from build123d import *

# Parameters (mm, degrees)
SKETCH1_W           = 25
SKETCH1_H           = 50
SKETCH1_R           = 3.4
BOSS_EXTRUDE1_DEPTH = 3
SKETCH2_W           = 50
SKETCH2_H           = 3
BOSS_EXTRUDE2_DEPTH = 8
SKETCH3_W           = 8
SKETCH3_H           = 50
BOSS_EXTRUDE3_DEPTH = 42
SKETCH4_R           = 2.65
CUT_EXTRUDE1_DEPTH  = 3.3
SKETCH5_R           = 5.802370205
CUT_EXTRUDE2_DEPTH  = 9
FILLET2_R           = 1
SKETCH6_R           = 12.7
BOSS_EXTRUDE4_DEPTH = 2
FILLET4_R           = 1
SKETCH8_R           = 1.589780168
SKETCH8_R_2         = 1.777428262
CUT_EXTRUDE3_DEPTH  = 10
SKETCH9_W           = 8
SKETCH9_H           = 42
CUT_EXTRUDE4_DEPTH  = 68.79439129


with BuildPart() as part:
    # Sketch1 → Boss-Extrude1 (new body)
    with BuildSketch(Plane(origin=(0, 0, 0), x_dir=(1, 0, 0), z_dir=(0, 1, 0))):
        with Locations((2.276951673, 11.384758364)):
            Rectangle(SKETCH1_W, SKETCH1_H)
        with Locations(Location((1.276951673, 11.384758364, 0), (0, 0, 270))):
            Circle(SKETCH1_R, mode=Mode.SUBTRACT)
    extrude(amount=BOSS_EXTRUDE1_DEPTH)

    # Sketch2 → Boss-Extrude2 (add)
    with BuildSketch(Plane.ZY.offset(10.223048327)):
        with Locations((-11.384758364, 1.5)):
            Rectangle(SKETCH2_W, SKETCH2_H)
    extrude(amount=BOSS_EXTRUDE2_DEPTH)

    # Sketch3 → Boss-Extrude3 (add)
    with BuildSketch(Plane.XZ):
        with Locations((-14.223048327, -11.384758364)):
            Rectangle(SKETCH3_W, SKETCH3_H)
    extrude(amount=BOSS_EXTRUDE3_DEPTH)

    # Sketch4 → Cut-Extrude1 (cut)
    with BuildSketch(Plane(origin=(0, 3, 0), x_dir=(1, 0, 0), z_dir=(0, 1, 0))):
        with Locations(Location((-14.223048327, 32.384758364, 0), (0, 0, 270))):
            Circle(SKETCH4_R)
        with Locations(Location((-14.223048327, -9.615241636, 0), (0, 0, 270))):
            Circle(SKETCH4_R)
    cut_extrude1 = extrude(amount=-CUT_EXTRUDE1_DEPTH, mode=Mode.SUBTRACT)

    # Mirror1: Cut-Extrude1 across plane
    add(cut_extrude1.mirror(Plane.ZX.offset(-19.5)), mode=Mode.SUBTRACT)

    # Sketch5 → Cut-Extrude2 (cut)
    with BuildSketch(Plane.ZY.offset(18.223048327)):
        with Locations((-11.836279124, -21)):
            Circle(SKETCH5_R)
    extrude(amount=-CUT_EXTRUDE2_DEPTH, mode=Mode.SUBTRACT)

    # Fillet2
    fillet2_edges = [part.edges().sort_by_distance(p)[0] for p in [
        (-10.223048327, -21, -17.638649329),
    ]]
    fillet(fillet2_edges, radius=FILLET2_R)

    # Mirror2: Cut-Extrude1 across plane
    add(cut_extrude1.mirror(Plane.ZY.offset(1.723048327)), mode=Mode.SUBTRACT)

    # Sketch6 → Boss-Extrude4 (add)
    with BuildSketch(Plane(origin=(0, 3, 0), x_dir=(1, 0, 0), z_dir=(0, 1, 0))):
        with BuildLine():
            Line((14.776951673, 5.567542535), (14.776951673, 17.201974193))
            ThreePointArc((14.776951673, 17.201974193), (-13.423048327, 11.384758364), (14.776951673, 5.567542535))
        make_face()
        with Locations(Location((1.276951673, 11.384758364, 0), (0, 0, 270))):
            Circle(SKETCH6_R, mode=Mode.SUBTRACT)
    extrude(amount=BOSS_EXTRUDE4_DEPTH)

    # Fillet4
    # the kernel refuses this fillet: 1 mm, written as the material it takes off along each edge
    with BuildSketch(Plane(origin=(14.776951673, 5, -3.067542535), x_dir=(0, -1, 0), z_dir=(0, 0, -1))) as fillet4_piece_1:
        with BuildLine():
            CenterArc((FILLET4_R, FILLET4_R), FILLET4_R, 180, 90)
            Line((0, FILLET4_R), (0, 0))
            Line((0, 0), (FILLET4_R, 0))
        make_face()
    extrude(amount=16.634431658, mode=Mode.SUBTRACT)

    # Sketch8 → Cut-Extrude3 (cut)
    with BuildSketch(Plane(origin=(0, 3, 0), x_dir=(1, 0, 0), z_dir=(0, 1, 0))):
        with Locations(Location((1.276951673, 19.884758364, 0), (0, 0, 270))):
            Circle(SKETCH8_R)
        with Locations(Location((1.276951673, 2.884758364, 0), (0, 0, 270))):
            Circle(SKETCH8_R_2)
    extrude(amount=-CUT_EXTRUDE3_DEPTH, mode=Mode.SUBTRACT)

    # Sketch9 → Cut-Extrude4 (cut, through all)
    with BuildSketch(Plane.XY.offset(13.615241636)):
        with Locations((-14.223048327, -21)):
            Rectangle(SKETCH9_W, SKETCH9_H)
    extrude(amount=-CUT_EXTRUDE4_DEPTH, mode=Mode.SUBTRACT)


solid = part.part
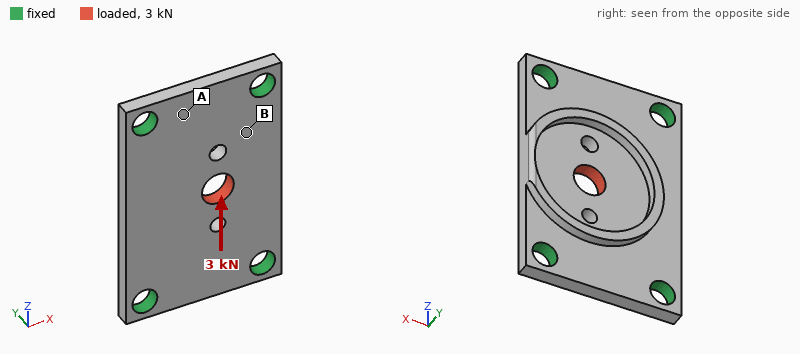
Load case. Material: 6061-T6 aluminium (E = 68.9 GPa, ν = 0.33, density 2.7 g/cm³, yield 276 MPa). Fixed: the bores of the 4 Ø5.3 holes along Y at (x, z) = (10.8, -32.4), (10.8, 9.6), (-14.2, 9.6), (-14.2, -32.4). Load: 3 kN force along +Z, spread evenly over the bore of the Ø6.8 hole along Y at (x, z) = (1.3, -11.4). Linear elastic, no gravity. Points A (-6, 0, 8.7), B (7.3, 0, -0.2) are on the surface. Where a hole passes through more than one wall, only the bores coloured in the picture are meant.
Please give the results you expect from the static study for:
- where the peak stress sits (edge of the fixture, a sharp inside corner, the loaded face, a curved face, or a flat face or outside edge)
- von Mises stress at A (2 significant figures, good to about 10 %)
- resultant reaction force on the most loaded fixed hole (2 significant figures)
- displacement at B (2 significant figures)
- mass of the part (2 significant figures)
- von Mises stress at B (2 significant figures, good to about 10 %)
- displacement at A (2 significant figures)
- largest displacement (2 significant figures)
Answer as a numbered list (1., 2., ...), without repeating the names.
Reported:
1. a curved face
2. 10 MPa
3. 890 N
4. 3.6 µm
5. 13 g
6. 32 MPa
7. 2.6 µm
8. 10 µm
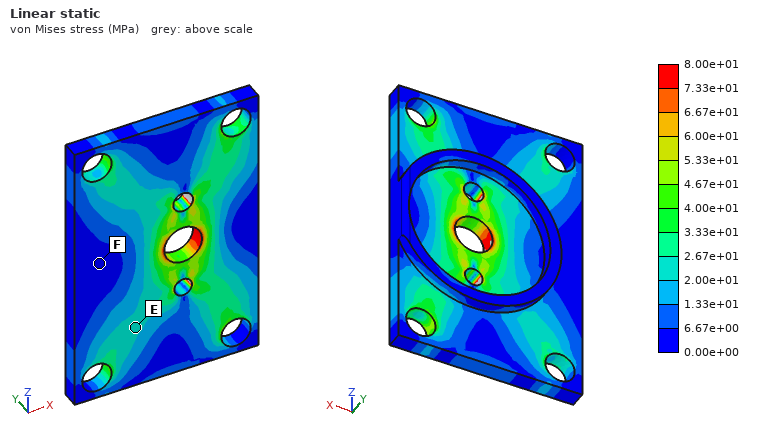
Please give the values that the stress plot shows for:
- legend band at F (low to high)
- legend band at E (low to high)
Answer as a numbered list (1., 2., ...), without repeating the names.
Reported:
1. 0.00e+00 to 6.67e+00 MPa
2. 2.00e+01 to 2.67e+01 MPa
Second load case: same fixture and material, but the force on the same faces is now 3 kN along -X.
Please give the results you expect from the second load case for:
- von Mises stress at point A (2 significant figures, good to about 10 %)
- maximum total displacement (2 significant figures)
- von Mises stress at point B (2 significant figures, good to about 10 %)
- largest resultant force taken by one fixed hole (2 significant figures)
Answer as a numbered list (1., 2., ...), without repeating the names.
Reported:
1. 16 MPa
2. 18 µm
3. 32 MPa
4. 980 N
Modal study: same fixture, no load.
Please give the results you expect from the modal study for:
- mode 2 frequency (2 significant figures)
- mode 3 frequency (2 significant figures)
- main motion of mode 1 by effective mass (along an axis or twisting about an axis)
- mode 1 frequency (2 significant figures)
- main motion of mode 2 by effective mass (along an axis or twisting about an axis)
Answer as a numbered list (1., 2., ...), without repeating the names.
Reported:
1. 13 kHz
2. 22 kHz
3. along Y
4. 9600 Hz
5. twisting about Z
